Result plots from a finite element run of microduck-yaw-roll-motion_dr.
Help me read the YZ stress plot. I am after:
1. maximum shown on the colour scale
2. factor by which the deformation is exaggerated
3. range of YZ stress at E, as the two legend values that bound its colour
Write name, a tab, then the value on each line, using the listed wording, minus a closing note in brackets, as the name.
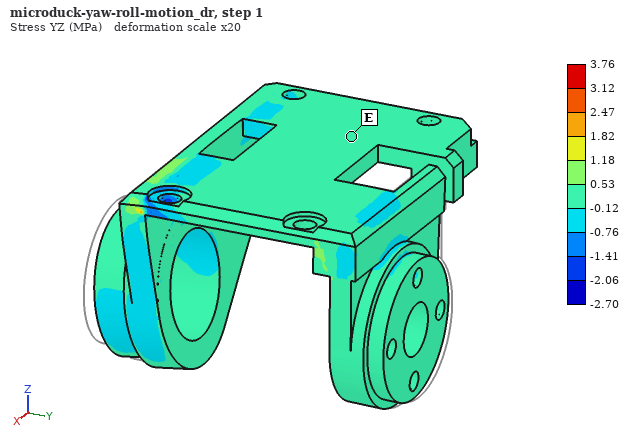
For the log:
maximum shown on the colour scale	3.76 MPa
factor by which the deformation is exaggerated	20
range of YZ stress at E, as the two legend values that bound its colour	-0.12 to 0.53 MPa
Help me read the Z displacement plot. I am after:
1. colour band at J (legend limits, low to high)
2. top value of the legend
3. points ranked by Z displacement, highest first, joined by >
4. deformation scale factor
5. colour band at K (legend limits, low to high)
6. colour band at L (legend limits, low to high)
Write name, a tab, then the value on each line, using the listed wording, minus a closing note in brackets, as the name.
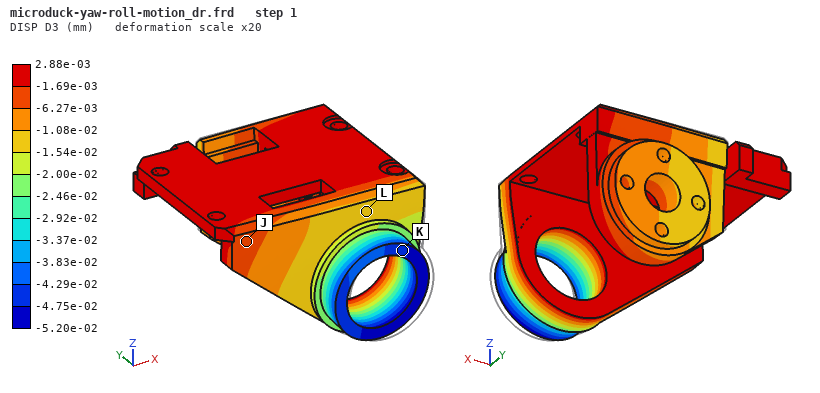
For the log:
colour band at J	-6.27e-03 to -1.69e-03 mm
top value of the legend	2.88e-03 mm
points ranked by Z displacement, highest first, joined by >	J > L > K
deformation scale factor	20
colour band at K	-4.75e-02 to -4.29e-02 mm
colour band at L	-1.54e-02 to -1.08e-02 mm
